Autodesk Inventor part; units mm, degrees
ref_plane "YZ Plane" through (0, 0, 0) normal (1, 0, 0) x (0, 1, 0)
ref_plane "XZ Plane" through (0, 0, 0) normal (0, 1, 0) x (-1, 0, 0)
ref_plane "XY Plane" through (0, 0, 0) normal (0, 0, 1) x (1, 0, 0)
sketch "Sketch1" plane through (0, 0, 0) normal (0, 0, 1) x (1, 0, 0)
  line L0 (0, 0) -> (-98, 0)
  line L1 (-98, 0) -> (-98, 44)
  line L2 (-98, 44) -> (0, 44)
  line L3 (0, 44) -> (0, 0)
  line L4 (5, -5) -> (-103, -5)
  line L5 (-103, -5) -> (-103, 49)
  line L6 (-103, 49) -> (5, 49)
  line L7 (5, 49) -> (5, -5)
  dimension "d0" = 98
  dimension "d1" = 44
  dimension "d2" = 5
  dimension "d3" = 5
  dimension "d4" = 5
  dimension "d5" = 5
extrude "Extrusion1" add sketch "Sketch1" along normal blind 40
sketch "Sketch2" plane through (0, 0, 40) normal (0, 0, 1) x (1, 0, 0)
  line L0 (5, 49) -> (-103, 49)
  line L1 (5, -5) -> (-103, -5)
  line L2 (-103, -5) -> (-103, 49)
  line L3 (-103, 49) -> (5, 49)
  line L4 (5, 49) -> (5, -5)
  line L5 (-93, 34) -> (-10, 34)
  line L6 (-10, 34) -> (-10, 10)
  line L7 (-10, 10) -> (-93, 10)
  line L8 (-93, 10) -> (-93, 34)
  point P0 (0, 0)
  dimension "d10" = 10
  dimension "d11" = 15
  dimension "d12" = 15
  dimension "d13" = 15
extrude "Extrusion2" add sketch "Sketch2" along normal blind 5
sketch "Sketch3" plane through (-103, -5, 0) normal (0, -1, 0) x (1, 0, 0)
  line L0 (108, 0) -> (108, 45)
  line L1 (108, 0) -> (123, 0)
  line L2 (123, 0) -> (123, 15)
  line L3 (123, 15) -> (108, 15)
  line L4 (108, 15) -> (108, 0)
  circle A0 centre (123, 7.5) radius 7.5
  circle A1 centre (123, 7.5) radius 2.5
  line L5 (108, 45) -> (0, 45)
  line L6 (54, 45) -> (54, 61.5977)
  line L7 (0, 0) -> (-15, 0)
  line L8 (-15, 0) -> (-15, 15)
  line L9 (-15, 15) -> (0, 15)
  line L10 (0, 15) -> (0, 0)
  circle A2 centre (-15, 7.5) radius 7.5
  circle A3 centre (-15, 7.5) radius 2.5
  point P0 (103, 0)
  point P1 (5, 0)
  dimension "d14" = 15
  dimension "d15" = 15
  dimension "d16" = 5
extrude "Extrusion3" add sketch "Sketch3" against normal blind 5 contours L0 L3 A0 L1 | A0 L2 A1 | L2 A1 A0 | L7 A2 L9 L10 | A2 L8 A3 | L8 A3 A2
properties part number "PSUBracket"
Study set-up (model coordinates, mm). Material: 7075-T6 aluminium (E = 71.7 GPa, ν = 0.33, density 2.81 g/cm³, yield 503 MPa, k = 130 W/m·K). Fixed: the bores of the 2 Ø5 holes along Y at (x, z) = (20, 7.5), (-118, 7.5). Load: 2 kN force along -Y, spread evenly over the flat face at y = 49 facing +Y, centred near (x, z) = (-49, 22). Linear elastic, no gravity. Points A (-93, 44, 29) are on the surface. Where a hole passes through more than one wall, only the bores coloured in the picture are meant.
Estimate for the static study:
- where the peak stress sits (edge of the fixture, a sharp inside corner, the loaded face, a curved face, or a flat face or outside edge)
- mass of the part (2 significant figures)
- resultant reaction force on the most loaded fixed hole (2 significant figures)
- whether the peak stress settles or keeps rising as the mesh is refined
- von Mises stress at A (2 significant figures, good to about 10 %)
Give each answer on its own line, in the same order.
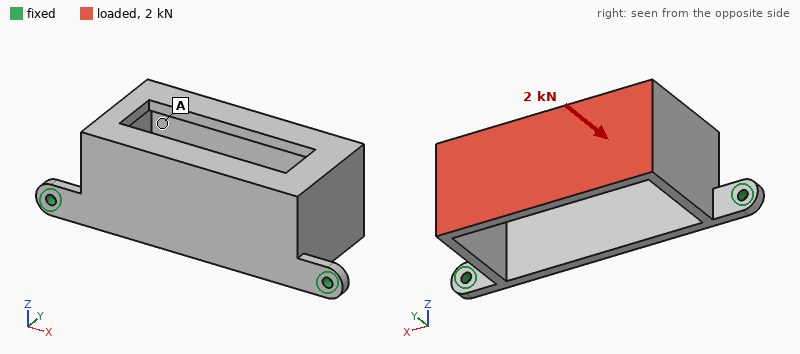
edge of the fixture
230 g
1.0 kN
keeps rising
22 MPa
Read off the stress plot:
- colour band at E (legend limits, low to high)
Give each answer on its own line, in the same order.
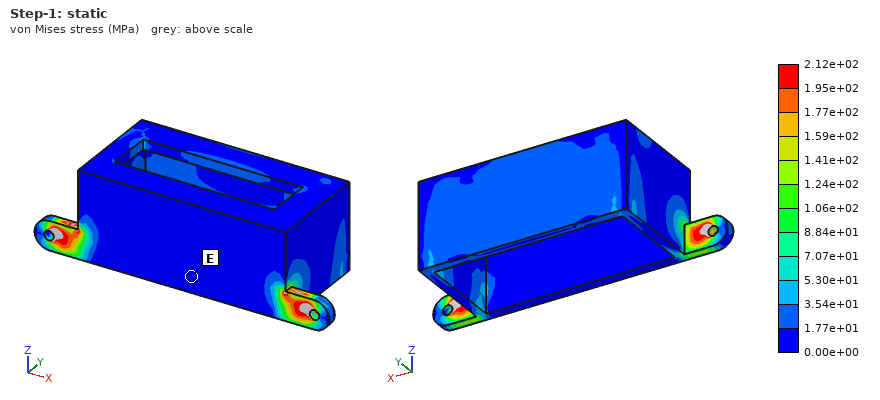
0.00e+00 to 1.77e+01 MPa
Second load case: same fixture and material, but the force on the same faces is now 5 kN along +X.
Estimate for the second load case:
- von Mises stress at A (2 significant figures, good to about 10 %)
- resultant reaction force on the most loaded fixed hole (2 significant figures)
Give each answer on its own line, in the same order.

78 MPa
3.3 kN
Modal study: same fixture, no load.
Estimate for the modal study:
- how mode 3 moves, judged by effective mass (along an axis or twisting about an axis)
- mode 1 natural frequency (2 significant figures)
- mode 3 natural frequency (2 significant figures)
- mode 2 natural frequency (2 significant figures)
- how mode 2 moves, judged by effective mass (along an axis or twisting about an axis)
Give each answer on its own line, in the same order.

along Y
380 Hz
1700 Hz
1000 Hz
along X
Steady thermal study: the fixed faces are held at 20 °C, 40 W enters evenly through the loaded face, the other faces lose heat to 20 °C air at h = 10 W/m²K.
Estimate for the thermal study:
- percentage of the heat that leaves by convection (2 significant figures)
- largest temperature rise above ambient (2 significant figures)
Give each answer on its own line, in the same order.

30 %
62 K
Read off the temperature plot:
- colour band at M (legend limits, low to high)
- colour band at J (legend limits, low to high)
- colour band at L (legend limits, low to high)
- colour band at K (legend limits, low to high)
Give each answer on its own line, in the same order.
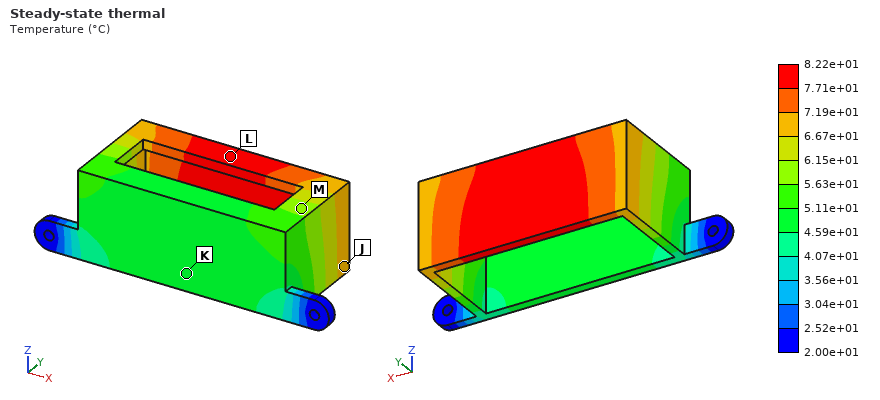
5.63e+01 to 6.15e+01 °C
6.67e+01 to 7.19e+01 °C
7.71e+01 to 8.22e+01 °C
4.59e+01 to 5.11e+01 °C
